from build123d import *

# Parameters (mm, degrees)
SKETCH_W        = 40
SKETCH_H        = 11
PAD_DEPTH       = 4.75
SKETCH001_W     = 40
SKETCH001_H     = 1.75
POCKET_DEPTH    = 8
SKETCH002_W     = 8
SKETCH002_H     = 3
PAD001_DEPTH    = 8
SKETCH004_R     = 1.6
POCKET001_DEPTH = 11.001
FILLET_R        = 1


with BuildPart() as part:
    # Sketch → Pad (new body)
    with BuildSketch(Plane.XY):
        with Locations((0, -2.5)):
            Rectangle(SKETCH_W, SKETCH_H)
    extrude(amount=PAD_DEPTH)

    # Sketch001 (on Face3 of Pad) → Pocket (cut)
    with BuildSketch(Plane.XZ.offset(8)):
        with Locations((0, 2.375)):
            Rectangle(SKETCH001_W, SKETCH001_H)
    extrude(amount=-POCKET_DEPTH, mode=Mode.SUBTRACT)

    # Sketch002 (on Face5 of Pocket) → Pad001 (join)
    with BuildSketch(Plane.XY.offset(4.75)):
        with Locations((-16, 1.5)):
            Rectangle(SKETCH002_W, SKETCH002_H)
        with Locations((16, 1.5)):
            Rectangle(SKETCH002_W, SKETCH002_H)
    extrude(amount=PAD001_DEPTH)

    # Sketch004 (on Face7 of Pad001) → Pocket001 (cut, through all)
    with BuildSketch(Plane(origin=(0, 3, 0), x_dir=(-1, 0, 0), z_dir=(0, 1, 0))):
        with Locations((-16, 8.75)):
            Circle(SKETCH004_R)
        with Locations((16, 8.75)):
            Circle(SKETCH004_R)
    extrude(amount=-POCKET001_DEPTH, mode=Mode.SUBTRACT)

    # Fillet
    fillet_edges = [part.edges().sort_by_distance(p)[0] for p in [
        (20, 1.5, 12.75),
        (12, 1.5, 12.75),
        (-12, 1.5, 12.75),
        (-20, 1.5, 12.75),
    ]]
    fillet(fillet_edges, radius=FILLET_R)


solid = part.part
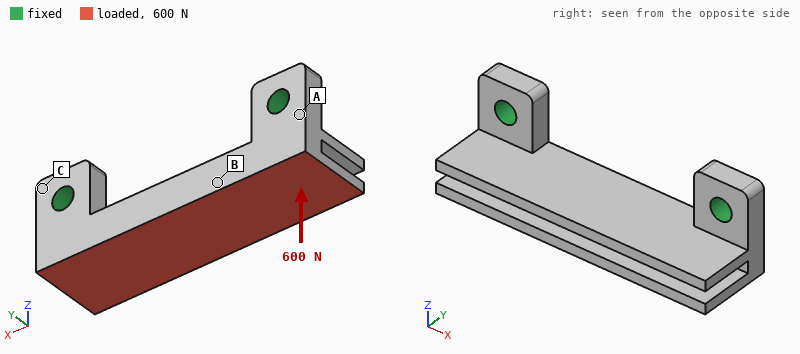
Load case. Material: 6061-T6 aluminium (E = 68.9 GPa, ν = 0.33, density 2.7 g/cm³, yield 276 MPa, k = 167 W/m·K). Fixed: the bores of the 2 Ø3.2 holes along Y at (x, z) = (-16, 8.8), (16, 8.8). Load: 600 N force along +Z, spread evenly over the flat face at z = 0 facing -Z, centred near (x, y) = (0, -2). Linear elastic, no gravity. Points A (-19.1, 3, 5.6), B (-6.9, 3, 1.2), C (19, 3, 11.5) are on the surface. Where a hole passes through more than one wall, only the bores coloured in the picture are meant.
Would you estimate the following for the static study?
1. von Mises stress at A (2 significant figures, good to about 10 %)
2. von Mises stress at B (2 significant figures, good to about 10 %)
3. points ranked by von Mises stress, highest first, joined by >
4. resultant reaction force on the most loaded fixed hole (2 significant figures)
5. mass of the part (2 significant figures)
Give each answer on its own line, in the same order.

78 MPa
26 MPa
A > B > C
330 N
5.0 g
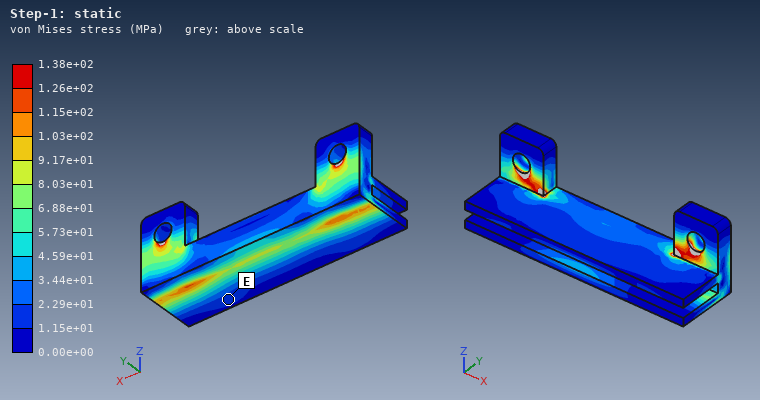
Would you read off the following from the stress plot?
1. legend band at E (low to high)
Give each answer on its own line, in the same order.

1.15e+01 to 2.29e+01 MPa
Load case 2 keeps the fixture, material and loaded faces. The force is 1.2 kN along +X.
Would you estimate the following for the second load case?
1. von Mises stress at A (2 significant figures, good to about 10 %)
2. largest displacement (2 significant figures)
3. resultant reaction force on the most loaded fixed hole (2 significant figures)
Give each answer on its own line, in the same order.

53 MPa
28 µm
630 N
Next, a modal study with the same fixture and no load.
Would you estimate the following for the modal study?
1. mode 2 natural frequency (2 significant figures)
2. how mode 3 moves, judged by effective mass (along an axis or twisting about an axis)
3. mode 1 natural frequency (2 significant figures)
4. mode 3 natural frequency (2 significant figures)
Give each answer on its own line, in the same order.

13 kHz
along Y
7700 Hz
16 kHz
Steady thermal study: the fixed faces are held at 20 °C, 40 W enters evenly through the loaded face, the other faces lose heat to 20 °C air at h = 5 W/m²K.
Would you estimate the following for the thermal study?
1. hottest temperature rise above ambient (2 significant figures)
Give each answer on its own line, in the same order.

55 K
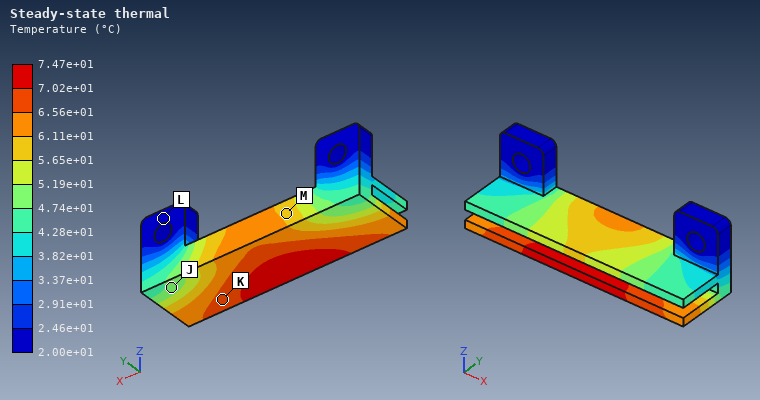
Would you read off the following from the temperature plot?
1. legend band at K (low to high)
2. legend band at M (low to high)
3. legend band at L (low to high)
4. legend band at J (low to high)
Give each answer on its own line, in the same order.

6.56e+01 to 7.02e+01 °C
5.65e+01 to 6.11e+01 °C
2.00e+01 to 2.46e+01 °C
4.74e+01 to 5.19e+01 °C
